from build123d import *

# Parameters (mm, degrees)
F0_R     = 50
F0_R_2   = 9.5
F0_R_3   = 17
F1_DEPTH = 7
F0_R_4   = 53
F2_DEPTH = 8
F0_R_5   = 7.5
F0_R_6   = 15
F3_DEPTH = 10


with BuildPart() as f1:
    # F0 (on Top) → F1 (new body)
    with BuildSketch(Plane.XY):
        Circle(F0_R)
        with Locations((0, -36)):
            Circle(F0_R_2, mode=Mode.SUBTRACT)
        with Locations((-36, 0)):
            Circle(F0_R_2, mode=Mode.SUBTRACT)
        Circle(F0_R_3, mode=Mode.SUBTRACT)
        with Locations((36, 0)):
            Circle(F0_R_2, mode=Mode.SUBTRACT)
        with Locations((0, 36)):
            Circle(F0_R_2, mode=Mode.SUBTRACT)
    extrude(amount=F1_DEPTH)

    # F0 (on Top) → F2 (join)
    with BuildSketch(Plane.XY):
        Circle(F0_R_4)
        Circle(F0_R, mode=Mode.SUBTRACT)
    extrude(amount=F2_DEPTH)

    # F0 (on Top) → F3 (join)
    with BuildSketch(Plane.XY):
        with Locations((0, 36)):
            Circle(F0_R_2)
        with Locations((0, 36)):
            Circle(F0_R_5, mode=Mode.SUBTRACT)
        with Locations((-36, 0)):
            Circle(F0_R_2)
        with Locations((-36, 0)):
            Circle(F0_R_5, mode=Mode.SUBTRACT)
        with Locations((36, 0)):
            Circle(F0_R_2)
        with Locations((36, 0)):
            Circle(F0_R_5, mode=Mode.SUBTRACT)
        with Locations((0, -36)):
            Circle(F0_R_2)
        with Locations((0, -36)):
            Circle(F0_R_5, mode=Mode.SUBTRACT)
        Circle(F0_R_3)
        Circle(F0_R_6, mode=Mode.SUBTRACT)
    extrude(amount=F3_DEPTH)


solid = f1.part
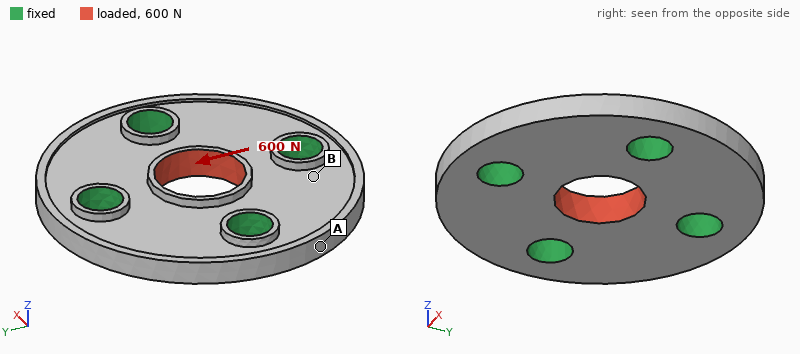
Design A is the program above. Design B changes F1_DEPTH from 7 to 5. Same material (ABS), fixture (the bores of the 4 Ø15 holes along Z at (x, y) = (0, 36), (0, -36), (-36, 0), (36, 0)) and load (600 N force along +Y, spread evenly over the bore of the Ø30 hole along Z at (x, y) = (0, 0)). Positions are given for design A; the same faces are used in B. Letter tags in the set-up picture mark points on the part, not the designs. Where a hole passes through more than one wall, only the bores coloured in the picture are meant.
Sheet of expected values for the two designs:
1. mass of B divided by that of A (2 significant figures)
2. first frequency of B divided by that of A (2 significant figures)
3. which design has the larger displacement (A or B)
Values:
0.79
0.76
B
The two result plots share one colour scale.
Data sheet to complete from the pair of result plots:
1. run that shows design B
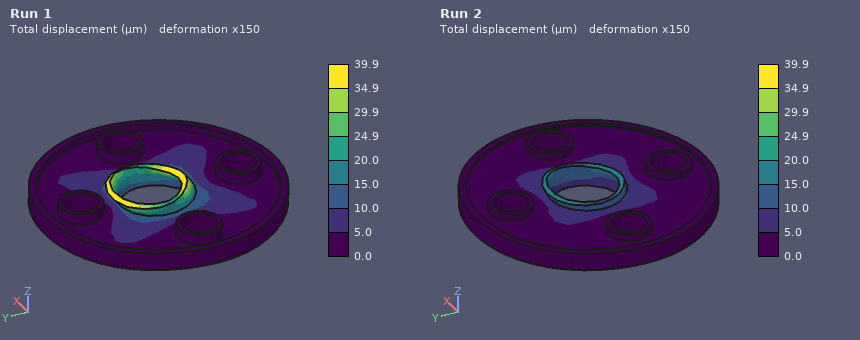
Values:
Run 1
